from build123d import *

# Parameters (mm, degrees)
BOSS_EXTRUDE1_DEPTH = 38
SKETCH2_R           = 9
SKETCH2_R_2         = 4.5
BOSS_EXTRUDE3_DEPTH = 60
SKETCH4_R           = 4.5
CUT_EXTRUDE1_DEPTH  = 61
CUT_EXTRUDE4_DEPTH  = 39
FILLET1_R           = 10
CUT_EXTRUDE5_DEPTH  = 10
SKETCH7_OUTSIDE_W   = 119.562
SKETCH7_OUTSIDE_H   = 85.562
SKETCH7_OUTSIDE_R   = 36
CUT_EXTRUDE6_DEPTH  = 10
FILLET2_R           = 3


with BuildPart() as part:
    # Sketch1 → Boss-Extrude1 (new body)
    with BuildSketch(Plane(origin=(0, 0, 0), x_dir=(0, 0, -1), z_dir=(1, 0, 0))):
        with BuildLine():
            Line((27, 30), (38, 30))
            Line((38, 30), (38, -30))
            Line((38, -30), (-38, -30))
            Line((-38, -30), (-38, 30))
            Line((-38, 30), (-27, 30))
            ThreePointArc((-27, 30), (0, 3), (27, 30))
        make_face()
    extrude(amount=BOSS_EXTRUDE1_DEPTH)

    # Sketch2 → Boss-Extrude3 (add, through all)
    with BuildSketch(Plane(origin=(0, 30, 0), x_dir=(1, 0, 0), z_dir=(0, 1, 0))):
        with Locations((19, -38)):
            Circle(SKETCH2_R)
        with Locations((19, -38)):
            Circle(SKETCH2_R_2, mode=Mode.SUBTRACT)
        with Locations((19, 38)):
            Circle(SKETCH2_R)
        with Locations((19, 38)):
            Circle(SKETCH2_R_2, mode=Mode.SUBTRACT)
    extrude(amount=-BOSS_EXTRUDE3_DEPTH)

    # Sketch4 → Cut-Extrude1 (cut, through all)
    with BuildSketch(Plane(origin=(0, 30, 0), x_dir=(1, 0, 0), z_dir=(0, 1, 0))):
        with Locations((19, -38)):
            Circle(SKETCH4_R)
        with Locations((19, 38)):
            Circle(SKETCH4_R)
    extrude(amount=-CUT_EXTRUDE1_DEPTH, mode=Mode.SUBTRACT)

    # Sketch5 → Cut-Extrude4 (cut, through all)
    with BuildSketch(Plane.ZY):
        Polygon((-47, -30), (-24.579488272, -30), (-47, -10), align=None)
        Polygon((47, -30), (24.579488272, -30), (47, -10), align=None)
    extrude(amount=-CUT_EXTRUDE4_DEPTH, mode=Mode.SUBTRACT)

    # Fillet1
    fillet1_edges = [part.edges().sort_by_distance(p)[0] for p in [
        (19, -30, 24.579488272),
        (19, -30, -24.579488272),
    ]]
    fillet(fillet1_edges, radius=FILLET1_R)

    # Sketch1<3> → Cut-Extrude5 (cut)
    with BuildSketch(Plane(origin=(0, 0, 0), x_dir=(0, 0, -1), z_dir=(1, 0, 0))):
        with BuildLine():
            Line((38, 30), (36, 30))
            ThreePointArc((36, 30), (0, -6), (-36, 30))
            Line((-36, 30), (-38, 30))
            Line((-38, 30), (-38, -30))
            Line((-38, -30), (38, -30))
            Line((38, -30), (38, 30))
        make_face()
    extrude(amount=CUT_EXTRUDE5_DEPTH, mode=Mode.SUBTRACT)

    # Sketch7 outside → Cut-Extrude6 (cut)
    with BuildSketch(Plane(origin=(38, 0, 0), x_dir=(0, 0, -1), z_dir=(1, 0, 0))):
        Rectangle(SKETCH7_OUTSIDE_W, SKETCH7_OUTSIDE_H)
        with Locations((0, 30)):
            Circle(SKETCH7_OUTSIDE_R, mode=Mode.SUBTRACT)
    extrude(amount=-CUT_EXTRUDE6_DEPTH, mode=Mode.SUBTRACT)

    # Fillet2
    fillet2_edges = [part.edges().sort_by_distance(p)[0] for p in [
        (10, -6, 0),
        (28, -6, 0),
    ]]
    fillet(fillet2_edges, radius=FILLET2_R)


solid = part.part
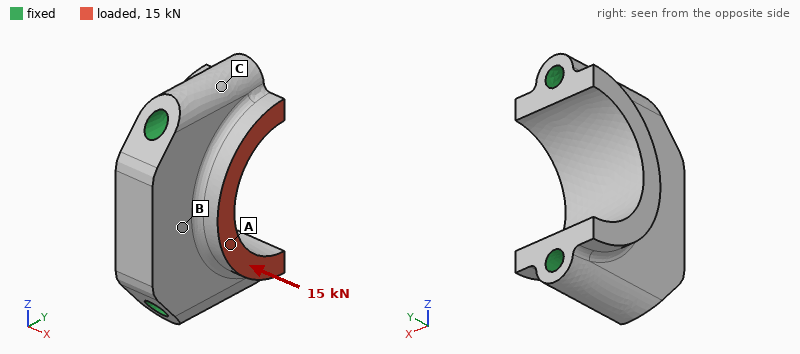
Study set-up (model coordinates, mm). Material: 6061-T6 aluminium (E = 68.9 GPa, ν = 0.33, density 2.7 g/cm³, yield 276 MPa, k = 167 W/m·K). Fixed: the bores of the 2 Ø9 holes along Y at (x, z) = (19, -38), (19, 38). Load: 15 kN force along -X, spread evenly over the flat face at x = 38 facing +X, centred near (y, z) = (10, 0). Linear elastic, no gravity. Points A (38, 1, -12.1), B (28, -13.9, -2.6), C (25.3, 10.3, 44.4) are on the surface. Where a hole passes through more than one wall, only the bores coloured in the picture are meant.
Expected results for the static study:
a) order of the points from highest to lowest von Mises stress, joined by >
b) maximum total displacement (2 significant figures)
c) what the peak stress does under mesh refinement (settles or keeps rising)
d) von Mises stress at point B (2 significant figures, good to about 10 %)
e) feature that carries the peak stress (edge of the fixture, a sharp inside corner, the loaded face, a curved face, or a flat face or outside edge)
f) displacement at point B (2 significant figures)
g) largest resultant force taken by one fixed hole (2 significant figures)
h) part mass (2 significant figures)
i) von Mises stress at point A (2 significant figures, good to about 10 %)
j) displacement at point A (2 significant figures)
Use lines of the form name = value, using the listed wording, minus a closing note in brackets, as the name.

order of the points from highest to lowest von Mises stress, joined by > = A > B > C
maximum total displacement = 15 µm
what the peak stress does under mesh refinement = keeps rising
von Mises stress at point B = 11 MPa
feature that carries the peak stress = edge of the fixture
displacement at point B = 11 µm
largest resultant force taken by one fixed hole = 7.5 kN
part mass = 220 g
von Mises stress at point A = 19 MPa
displacement at point A = 14 µm
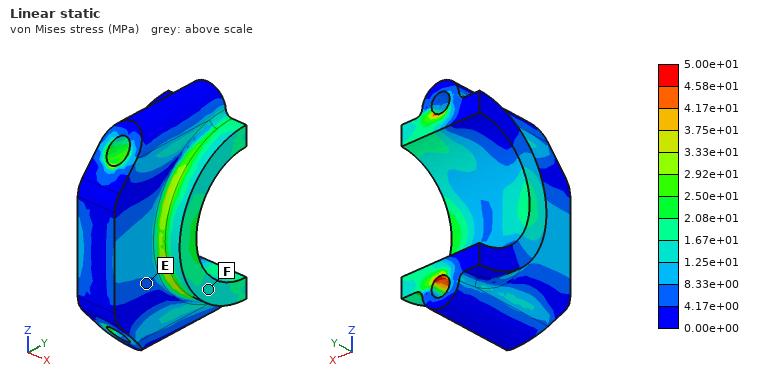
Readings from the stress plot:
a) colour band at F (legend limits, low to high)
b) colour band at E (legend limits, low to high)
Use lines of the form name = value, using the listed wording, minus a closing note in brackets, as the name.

colour band at F = 1.25e+01 to 1.67e+01 MPa
colour band at E = 4.17e+00 to 8.33e+00 MPa
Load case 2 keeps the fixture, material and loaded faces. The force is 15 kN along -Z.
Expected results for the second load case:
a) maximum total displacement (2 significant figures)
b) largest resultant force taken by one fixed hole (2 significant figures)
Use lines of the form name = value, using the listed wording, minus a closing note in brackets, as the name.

maximum total displacement = 38 µm
largest resultant force taken by one fixed hole = 8.1 kN
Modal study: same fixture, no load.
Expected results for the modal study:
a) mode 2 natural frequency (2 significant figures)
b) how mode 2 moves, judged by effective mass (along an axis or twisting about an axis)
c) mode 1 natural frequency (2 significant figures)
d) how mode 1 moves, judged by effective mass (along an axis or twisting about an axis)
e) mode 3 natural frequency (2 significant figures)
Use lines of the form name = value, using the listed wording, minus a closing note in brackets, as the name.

mode 2 natural frequency = 19 kHz
how mode 2 moves, judged by effective mass = along Y
mode 1 natural frequency = 12 kHz
how mode 1 moves, judged by effective mass = along X
mode 3 natural frequency = 20 kHz
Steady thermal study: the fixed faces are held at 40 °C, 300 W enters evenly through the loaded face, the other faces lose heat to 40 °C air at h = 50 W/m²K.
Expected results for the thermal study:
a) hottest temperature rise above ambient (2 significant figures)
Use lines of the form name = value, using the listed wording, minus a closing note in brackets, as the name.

hottest temperature rise above ambient = 43 K
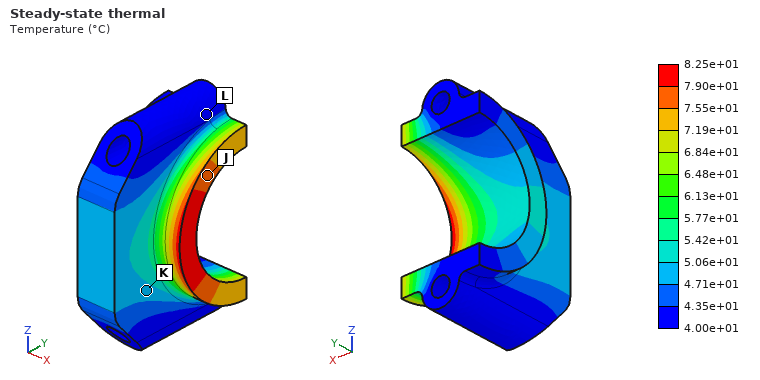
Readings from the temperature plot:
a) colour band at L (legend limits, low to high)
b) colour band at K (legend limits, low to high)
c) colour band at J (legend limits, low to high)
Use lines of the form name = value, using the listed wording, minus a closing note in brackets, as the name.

colour band at L = 4.00e+01 to 4.35e+01 °C
colour band at K = 4.71e+01 to 5.06e+01 °C
colour band at J = 7.55e+01 to 7.90e+01 °C
